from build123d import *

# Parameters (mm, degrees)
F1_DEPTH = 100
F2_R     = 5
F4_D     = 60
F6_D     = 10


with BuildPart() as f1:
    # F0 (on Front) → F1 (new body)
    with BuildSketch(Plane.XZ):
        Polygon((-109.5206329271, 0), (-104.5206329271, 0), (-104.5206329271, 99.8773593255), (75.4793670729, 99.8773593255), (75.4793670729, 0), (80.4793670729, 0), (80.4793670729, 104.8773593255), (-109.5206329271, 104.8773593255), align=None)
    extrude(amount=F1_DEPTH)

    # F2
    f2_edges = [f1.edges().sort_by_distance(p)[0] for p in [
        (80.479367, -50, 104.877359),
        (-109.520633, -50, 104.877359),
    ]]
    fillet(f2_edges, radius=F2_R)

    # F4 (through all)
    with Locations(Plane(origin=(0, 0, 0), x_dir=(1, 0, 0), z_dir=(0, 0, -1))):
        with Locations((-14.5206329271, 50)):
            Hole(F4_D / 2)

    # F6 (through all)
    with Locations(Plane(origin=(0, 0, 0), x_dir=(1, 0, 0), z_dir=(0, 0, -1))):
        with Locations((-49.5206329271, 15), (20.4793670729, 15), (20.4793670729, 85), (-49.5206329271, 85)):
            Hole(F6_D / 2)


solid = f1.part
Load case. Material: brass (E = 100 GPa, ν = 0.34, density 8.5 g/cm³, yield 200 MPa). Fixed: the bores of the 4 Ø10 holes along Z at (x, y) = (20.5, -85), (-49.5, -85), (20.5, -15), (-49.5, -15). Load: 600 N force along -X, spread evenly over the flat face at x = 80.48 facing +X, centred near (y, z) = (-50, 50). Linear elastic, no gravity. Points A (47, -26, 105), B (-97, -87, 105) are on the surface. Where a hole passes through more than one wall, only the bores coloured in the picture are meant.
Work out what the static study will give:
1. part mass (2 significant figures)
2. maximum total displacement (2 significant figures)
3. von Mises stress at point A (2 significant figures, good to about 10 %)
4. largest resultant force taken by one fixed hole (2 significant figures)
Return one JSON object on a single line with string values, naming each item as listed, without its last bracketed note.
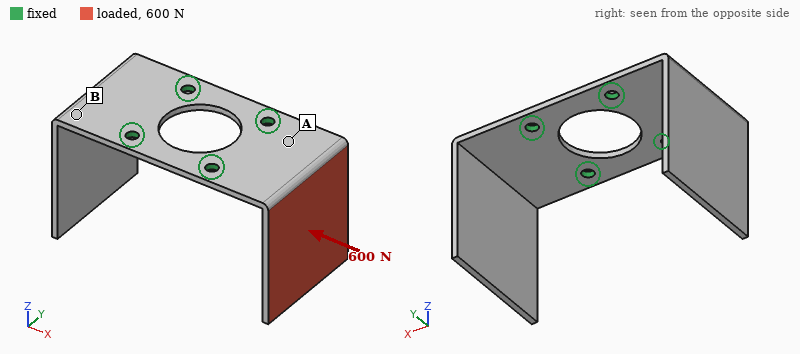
{"part mass": "1.5 kg", "maximum total displacement": "2.4 mm", "von Mises stress at point A": "65 MPa", "largest resultant force taken by one fixed hole": "320 N"}
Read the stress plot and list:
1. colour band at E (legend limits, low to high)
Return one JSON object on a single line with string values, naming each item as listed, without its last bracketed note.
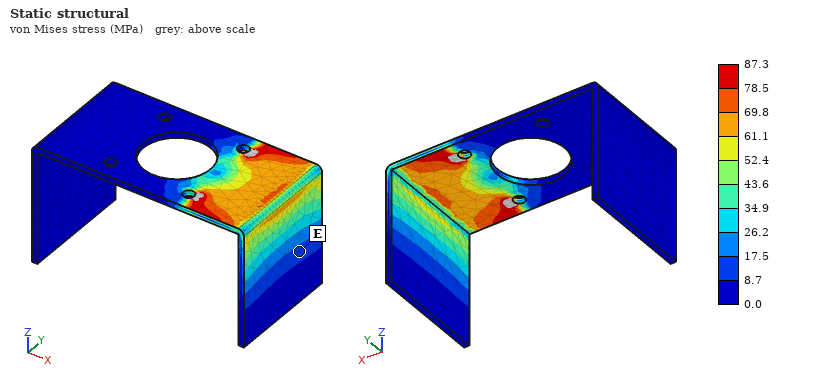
{"colour band at E": "8.7 to 17.5 MPa"}
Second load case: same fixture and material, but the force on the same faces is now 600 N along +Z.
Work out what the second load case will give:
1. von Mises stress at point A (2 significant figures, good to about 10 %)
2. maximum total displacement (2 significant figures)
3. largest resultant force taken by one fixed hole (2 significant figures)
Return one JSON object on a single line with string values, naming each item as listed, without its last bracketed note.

{"von Mises stress at point A": "42 MPa", "maximum total displacement": "1.1 mm", "largest resultant force taken by one fixed hole": "310 N"}
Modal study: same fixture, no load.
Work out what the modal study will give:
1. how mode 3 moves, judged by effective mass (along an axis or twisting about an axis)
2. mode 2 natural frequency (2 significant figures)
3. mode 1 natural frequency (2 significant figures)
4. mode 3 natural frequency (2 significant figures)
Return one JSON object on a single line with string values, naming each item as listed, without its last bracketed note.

{"how mode 3 moves, judged by effective mass": "along Y", "mode 2 natural frequency": "140 Hz", "mode 1 natural frequency": "140 Hz", "mode 3 natural frequency": "290 Hz"}
